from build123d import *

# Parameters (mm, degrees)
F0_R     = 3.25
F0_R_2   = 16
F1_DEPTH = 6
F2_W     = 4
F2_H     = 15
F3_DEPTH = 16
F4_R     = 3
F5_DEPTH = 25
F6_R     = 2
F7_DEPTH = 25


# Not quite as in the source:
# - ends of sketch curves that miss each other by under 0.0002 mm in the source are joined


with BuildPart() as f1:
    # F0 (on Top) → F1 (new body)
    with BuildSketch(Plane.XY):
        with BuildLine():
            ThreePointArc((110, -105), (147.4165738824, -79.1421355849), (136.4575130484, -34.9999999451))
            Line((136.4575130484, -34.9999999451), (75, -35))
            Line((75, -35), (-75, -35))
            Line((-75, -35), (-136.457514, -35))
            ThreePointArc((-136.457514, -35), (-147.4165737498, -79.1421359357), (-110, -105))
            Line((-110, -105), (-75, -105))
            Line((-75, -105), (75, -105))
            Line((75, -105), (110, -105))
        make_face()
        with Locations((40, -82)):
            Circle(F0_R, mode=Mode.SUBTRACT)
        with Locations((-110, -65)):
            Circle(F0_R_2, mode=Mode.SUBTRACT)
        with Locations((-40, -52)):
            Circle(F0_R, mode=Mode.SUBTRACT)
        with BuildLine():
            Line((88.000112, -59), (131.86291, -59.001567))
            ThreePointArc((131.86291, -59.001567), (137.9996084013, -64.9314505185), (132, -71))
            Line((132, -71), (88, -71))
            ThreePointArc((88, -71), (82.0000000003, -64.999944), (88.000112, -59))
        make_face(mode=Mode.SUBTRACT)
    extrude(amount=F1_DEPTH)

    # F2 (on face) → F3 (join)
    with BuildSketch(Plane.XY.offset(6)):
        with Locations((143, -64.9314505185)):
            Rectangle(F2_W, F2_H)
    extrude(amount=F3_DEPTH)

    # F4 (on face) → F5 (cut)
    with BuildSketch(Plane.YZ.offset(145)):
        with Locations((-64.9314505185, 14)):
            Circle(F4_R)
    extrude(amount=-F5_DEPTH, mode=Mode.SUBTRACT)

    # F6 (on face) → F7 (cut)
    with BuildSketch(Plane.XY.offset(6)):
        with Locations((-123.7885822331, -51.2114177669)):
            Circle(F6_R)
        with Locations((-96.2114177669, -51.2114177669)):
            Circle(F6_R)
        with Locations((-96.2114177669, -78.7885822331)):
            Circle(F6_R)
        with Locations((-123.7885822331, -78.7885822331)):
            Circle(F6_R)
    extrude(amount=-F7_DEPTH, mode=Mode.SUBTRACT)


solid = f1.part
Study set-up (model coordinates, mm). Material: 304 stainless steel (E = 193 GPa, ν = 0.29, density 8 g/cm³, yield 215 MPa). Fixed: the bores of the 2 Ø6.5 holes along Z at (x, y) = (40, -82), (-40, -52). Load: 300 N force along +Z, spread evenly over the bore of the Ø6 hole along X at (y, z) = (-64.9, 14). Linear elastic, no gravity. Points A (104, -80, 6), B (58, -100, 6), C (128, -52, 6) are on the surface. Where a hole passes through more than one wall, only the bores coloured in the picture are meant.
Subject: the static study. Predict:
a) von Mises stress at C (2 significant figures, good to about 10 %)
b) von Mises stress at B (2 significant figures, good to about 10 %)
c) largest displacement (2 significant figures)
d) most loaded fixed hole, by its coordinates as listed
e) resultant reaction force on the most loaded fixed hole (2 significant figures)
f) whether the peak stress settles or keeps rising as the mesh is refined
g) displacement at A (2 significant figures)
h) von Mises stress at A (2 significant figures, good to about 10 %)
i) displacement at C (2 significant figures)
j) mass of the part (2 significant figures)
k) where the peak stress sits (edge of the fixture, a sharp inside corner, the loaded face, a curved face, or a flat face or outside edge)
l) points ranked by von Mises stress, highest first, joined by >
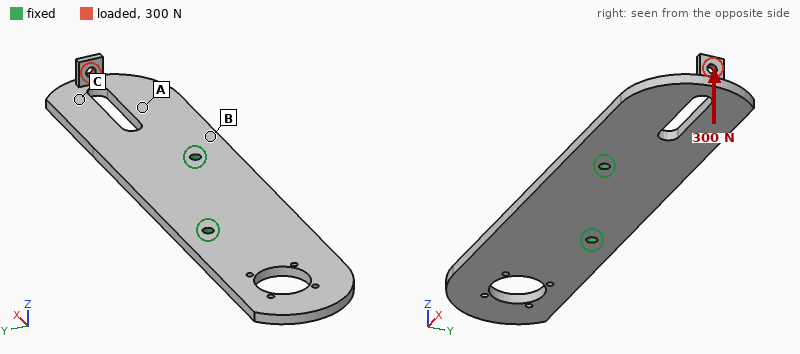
14 MPa
67 MPa
0.59 mm
(40, -82)
430 N
keeps rising
0.24 mm
35 MPa
0.43 mm
890 g
edge of the fixture
B > A > C
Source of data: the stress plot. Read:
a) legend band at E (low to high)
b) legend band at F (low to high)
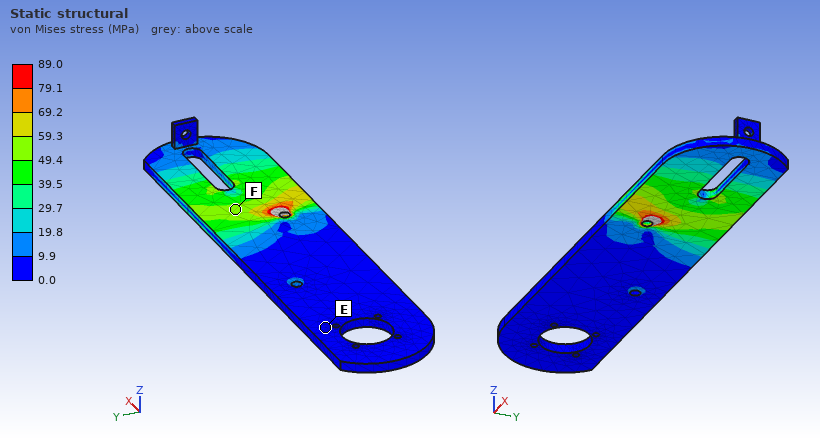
0.0 to 9.9 MPa
49.4 to 59.3 MPa
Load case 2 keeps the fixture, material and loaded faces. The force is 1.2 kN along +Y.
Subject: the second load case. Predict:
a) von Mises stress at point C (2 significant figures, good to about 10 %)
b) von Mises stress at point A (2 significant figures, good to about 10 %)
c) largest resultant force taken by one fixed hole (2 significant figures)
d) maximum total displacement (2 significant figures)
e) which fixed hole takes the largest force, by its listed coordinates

50 MPa
38 MPa
2.5 kN
0.19 mm
(40, -82)
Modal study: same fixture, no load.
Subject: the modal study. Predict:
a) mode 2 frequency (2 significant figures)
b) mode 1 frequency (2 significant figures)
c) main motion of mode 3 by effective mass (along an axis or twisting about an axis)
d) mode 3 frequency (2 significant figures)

420 Hz
410 Hz
twisting about X
1100 Hz
